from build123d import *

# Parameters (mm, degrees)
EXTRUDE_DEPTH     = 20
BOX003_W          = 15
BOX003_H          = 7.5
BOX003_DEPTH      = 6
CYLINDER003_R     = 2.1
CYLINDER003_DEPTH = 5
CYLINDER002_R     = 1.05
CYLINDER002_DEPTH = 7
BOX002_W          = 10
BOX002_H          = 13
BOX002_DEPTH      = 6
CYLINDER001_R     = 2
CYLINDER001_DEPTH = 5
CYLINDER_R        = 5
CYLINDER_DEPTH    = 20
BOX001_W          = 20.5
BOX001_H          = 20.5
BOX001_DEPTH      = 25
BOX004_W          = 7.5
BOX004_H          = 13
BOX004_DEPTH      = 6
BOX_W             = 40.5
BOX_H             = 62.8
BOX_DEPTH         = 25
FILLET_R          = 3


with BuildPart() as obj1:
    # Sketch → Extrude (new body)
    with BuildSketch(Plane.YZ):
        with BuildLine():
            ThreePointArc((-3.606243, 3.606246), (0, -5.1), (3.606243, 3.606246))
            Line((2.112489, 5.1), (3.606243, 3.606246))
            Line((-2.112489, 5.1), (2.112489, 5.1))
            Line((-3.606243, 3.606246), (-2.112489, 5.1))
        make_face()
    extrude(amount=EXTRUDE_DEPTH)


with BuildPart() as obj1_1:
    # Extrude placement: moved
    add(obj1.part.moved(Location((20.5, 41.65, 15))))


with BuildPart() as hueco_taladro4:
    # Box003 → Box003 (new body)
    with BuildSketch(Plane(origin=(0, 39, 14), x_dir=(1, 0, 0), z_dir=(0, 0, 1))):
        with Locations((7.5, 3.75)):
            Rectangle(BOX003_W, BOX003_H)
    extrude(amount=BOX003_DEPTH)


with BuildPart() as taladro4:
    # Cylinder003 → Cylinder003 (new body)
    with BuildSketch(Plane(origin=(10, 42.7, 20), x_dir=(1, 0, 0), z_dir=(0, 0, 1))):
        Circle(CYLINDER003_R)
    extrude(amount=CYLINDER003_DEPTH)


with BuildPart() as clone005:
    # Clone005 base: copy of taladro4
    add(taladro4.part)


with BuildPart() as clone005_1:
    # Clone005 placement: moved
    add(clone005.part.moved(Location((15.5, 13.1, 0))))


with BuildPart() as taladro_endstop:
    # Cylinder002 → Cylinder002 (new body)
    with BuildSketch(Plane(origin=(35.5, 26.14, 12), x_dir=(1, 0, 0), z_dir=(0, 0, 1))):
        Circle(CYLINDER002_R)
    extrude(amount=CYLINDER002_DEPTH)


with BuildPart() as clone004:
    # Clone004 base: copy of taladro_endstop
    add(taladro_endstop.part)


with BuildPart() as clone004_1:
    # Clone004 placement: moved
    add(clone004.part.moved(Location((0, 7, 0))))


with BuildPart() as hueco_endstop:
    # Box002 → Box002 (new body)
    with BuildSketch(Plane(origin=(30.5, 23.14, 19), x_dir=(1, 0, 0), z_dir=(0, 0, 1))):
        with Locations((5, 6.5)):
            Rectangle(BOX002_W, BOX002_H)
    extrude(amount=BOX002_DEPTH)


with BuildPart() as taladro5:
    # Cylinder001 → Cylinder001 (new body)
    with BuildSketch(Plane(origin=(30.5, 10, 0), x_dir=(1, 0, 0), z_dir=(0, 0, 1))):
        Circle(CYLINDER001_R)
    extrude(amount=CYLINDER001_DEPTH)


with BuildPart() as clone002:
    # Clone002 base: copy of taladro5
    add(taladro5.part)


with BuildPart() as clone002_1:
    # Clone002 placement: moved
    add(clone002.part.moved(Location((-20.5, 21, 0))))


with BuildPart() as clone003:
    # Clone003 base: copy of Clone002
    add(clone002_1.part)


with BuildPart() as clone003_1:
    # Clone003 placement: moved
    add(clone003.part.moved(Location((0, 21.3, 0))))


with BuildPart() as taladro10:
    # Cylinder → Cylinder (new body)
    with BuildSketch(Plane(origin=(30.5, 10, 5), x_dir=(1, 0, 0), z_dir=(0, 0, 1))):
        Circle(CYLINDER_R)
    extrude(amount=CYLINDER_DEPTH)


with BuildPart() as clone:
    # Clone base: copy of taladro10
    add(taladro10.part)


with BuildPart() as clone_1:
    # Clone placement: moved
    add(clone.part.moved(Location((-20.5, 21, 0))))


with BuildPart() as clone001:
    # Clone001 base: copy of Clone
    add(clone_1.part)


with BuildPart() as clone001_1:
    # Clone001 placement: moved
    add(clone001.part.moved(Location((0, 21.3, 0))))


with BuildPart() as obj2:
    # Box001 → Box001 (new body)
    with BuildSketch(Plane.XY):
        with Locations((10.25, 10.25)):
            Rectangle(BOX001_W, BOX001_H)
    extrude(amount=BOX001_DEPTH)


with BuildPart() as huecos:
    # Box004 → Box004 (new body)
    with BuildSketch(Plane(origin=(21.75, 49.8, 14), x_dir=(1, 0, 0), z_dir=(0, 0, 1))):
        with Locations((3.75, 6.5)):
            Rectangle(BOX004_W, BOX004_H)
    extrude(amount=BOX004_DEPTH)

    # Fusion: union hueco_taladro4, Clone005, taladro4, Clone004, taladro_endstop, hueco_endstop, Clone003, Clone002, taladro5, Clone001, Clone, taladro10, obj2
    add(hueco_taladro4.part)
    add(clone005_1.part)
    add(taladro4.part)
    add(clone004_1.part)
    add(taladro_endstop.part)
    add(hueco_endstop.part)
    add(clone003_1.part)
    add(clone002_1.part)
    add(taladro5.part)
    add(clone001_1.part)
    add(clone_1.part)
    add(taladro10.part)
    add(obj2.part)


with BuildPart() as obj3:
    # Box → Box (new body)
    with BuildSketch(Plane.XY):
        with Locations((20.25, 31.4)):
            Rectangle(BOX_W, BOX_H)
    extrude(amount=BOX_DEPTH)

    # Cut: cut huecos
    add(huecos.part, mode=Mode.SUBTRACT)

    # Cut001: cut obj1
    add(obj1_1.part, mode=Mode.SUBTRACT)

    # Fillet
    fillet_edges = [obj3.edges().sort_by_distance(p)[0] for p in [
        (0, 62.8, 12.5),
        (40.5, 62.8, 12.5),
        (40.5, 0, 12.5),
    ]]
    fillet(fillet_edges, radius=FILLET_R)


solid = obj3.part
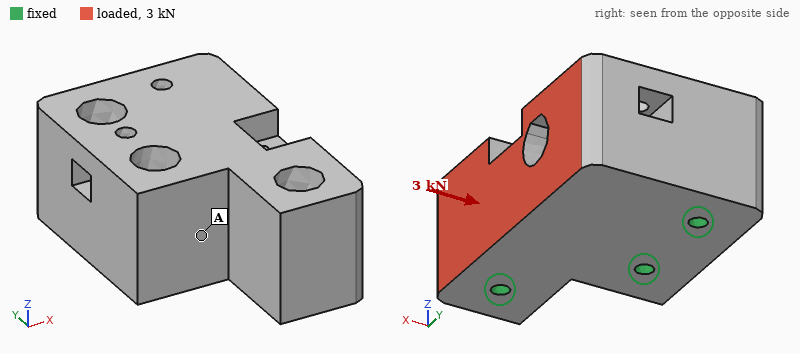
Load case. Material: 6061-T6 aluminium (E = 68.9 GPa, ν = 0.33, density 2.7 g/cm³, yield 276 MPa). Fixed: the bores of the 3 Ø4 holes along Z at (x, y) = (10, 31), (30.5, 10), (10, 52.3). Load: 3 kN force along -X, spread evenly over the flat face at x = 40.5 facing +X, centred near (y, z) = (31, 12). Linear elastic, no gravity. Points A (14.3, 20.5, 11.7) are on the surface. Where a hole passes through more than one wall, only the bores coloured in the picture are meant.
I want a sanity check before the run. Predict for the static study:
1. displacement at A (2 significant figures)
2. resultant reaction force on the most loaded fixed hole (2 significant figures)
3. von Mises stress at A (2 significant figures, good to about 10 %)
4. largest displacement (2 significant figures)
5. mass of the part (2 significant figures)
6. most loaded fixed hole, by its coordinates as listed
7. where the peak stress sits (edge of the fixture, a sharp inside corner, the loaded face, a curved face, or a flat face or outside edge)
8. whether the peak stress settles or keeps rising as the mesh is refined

9.2 µm
1.7 kN
8.8 MPa
33 µm
120 g
(10, 31)
edge of the fixture
keeps rising
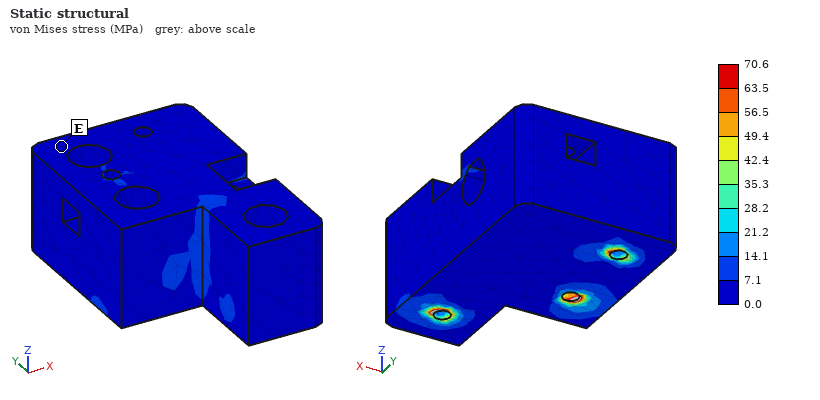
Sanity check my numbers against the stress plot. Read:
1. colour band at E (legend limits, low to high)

0.0 to 7.1 MPa
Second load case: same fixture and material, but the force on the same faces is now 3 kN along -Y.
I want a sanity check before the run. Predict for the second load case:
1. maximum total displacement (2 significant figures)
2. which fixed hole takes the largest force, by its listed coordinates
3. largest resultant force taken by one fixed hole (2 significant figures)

19 µm
(30.5, 10)
2.2 kN
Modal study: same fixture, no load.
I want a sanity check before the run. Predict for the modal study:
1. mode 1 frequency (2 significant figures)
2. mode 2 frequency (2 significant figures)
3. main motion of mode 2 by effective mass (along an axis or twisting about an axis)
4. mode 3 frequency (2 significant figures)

4500 Hz
12 kHz
along Y
13 kHz
